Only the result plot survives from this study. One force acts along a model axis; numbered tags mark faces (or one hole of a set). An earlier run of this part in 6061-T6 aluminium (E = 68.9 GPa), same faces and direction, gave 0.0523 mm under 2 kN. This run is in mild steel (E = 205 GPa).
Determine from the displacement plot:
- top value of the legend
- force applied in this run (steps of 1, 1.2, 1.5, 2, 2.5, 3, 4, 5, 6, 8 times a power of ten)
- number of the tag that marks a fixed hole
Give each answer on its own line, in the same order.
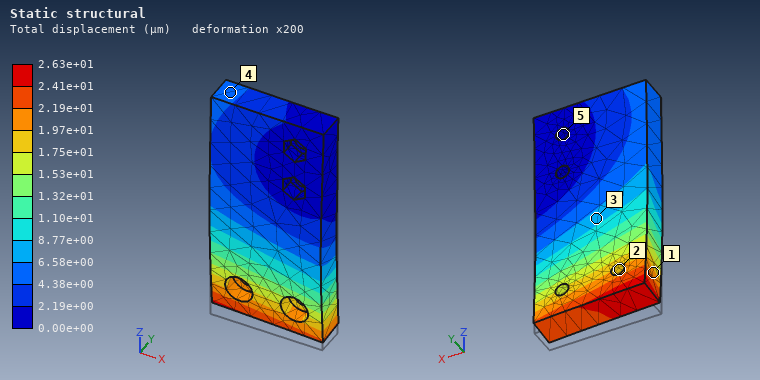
2.63e+01 µm
3 kN
5
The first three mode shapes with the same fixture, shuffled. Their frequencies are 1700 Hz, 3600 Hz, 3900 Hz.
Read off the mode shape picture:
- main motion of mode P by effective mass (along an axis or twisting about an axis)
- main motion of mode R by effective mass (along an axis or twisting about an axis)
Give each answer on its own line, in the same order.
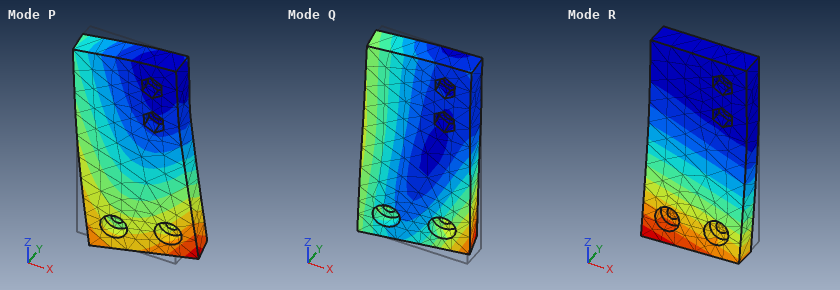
along X
along Y
